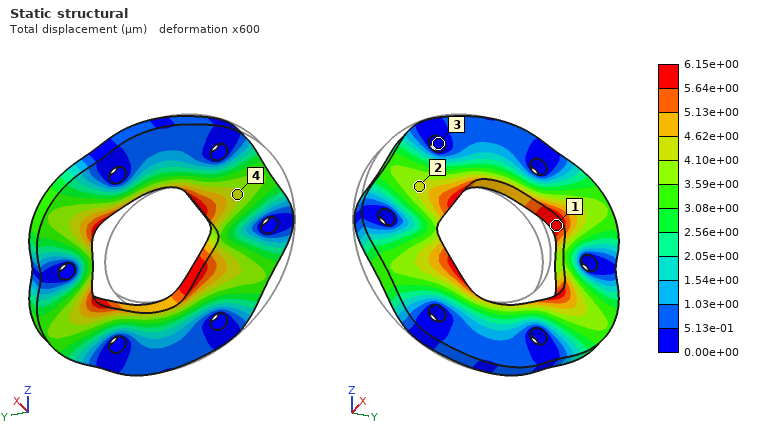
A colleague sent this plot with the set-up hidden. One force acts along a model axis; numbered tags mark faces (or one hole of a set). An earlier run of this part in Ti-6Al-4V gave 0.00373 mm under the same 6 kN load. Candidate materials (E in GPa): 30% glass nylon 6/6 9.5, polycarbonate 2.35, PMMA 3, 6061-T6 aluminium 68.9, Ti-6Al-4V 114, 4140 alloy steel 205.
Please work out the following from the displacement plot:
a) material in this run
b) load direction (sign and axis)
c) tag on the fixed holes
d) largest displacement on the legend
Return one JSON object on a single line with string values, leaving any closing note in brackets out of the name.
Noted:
{"material in this run": "6061-T6 aluminium", "load direction": "+Y", "tag on the fixed holes": "3", "largest displacement on the legend": "6.15e+00 µm"}
